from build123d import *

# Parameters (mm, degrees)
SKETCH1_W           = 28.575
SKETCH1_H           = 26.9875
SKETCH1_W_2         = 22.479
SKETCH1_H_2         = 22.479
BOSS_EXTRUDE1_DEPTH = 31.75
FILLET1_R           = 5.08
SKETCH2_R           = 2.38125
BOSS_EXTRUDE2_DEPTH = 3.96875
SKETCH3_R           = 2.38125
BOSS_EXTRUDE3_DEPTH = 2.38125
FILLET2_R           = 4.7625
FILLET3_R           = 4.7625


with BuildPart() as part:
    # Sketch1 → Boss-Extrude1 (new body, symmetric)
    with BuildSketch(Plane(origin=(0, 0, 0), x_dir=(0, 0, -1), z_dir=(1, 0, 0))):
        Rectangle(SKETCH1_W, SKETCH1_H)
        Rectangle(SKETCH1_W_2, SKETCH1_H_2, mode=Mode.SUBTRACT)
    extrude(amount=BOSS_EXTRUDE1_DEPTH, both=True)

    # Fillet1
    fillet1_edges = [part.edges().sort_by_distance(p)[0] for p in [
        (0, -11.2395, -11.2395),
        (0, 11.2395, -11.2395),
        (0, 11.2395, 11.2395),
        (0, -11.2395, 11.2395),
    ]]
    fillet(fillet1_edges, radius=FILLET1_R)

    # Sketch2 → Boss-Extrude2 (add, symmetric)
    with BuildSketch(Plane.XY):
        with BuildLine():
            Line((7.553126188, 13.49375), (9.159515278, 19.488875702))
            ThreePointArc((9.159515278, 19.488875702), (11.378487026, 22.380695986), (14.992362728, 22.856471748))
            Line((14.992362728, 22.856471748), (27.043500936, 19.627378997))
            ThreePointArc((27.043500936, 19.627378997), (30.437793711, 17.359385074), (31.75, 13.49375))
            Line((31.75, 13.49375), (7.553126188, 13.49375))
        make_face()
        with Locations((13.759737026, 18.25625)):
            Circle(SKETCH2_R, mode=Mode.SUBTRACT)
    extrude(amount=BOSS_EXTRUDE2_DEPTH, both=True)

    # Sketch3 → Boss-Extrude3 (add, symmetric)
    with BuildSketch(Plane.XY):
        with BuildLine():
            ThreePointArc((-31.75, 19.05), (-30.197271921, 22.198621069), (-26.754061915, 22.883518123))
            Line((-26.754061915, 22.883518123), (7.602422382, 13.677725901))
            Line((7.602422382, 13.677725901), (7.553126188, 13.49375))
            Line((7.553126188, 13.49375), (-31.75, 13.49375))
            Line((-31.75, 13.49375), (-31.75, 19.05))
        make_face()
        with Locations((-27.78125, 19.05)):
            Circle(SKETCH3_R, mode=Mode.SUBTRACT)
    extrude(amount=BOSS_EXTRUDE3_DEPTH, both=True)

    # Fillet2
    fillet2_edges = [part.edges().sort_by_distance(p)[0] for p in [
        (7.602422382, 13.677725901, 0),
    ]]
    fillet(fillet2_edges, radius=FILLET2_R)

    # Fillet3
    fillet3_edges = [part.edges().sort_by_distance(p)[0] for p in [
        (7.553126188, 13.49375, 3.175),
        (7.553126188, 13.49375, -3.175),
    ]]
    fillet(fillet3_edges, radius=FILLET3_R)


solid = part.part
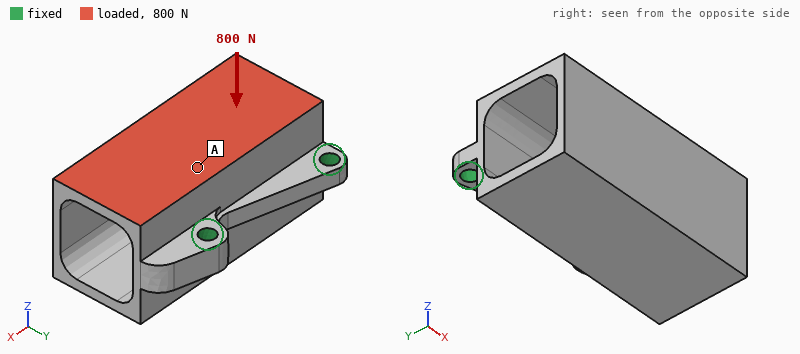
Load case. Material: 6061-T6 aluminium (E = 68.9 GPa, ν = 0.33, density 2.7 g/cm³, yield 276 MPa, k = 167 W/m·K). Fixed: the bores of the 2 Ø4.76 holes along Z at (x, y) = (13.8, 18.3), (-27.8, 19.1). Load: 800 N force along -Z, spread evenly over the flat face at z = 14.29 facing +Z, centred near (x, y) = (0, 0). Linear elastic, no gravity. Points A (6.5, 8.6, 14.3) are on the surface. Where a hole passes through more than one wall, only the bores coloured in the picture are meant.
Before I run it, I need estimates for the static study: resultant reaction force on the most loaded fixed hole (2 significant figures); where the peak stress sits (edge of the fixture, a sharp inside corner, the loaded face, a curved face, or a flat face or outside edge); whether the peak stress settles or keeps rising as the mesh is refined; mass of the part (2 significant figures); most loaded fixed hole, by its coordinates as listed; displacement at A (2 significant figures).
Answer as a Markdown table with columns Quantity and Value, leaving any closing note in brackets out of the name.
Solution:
| Quantity | Value |
|---|---|
| resultant reaction force on the most loaded fixed hole | 580 N |
| where the peak stress sits | edge of the fixture |
| whether the peak stress settles or keeps rising as the mesh is refined | keeps rising |
| mass of the part | 55 g |
| most loaded fixed hole, by its coordinates as listed | (13.8, 18.3) |
| displacement at A | 0.090 mm |
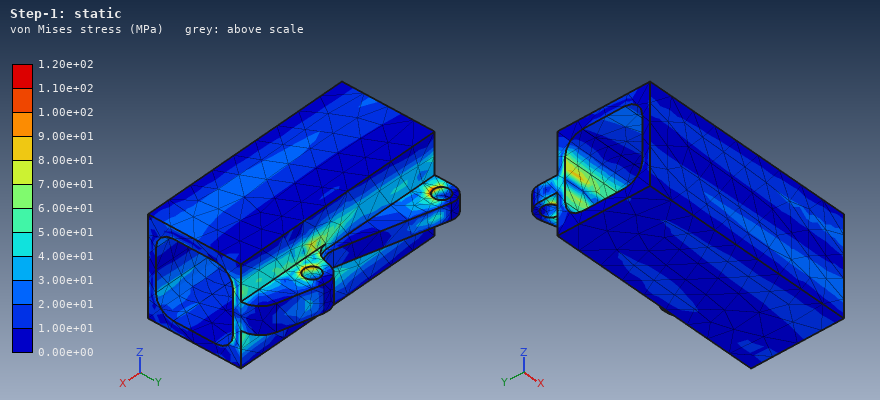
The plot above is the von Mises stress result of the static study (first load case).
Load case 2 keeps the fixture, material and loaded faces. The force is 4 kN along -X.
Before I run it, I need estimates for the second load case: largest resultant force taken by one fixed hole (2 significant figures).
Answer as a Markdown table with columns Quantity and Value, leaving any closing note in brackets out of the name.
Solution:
| Quantity | Value |
|---|---|
| largest resultant force taken by one fixed hole | 2.8 kN |
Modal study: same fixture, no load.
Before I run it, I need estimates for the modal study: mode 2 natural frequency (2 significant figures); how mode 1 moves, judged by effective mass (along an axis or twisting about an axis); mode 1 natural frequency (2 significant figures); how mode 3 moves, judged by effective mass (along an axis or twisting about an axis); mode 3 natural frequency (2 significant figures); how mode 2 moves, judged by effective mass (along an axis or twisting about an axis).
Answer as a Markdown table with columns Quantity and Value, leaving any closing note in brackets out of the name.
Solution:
| Quantity | Value |
|---|---|
| mode 2 natural frequency | 4600 Hz |
| how mode 1 moves, judged by effective mass | along Z |
| mode 1 natural frequency | 1500 Hz |
| how mode 3 moves, judged by effective mass | along Y |
| mode 3 natural frequency | 5600 Hz |
| how mode 2 moves, judged by effective mass | along X |
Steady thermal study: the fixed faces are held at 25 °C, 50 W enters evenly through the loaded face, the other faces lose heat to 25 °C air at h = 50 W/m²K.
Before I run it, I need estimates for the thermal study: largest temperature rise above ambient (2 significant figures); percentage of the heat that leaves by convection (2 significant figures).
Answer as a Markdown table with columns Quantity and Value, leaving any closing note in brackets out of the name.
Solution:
| Quantity | Value |
|---|---|
| largest temperature rise above ambient | 29 K |
| percentage of the heat that leaves by convection | 19 % |
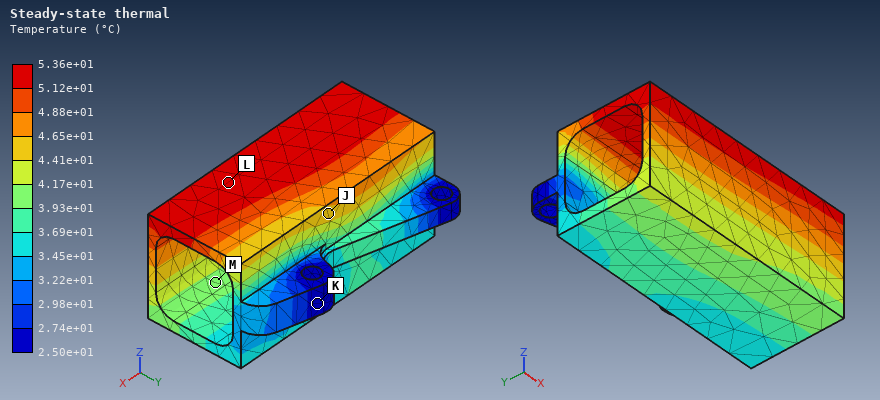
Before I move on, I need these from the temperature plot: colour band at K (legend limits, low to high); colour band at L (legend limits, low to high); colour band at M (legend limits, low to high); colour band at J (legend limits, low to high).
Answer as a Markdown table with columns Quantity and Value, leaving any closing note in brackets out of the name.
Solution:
| Quantity | Value |
|---|---|
| colour band at K | 2.50e+01 to 2.74e+01 °C |
| colour band at L | 5.12e+01 to 5.36e+01 °C |
| colour band at M | 3.93e+01 to 4.17e+01 °C |
| colour band at J | 4.41e+01 to 4.65e+01 °C |
